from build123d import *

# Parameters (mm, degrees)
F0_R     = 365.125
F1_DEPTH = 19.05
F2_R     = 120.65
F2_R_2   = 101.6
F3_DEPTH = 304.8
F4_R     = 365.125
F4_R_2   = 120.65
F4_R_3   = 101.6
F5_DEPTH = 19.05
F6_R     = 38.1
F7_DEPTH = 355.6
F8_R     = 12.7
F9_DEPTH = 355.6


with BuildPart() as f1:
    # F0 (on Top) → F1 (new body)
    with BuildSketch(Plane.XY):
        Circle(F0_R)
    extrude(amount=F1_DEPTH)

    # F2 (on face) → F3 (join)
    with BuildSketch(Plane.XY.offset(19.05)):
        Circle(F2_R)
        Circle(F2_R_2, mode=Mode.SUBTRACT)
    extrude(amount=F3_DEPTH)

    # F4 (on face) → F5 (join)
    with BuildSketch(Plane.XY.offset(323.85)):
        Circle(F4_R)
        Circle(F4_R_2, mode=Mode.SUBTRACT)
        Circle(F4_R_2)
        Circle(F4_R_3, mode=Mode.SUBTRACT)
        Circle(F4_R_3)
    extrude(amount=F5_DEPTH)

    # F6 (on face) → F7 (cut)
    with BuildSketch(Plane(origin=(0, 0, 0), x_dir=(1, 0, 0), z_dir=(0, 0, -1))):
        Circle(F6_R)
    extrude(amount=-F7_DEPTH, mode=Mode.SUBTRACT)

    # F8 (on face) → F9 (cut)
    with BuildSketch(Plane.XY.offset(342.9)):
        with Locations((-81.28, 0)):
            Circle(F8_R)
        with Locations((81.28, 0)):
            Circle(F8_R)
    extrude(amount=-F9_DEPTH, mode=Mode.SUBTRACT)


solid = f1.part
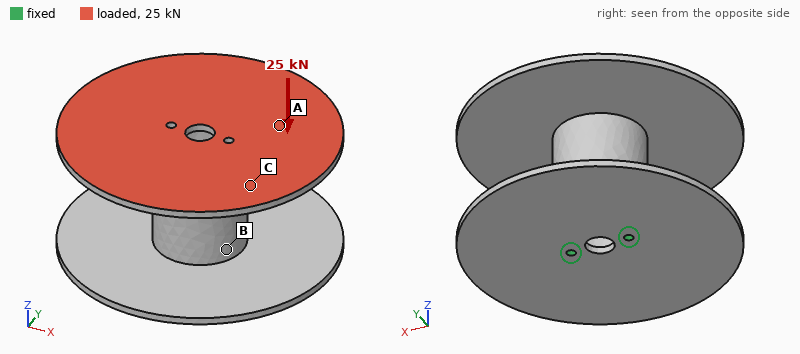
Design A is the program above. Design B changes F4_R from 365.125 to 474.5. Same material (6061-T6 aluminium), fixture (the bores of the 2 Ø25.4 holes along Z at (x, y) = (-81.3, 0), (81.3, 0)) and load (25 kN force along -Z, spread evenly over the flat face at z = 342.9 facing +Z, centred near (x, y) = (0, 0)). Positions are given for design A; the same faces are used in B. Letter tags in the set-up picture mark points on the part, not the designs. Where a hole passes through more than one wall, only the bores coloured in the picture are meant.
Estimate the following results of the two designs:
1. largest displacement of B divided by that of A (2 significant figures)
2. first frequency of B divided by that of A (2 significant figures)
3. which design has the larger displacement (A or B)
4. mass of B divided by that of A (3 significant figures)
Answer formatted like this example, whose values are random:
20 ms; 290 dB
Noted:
2.3; 0.75; B; 1.28
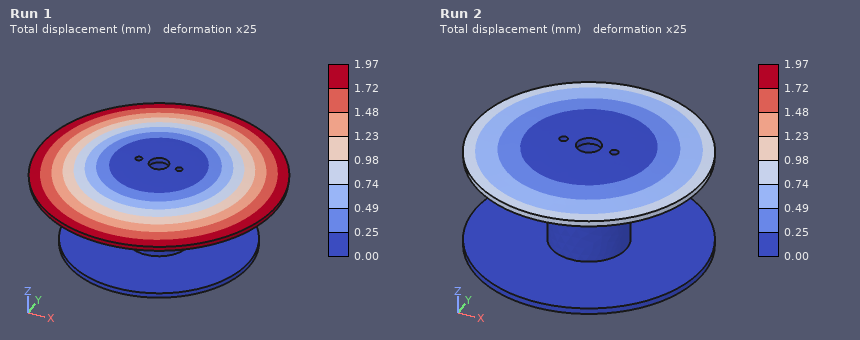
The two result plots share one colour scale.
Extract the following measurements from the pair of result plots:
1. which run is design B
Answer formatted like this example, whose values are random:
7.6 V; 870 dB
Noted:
Run 1
